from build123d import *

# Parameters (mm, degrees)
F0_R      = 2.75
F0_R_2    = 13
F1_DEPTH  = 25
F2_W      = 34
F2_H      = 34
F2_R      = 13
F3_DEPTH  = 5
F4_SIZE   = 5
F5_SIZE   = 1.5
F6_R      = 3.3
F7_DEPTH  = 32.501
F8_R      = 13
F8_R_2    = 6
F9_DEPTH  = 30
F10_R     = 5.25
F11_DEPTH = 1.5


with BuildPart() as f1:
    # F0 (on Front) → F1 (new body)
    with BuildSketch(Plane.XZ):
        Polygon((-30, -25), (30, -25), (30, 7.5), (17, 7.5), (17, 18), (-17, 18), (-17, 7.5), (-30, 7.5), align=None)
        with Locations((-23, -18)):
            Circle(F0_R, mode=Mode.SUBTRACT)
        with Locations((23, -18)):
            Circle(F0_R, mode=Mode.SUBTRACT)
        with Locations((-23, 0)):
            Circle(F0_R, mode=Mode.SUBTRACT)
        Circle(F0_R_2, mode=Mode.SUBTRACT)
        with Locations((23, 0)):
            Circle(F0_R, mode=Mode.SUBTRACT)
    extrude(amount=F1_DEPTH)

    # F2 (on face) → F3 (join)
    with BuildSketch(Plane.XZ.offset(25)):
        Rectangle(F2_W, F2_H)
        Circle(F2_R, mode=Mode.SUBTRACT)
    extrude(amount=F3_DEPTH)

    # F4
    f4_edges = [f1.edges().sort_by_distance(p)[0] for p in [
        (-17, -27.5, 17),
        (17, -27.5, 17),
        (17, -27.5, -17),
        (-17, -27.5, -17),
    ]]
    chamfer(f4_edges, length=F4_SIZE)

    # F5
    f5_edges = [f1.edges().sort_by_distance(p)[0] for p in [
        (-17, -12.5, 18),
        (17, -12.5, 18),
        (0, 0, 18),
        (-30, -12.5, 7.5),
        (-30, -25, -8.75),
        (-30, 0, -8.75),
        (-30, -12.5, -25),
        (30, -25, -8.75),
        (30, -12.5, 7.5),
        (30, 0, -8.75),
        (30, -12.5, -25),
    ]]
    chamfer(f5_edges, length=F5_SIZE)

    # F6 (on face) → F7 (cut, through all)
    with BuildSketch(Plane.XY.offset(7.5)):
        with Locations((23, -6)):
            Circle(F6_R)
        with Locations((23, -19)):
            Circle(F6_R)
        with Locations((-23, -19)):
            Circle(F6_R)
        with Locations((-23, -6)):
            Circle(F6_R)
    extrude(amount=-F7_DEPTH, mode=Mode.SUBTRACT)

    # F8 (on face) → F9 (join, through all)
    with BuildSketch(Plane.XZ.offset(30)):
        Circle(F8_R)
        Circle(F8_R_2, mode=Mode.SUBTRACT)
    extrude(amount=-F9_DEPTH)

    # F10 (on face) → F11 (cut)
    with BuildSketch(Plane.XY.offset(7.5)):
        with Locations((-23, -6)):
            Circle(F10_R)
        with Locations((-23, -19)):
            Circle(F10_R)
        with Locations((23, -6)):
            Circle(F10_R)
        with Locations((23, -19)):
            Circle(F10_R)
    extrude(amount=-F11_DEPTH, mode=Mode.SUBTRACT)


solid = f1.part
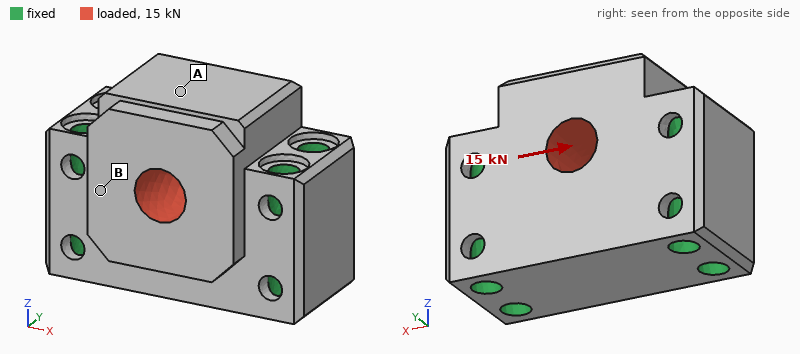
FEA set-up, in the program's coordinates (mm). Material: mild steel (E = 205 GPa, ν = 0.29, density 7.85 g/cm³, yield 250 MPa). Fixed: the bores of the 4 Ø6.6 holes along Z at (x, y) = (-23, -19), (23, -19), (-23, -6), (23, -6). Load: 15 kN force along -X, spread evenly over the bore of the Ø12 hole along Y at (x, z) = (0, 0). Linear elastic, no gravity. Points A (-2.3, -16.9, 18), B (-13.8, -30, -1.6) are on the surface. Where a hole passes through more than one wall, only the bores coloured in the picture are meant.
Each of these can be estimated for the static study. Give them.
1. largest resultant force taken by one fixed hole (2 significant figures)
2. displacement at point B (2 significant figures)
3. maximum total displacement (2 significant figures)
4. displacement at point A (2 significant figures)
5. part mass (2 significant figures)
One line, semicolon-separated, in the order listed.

4.2 kN; 1.1 µm; 1.8 µm; 0.99 µm; 420 g
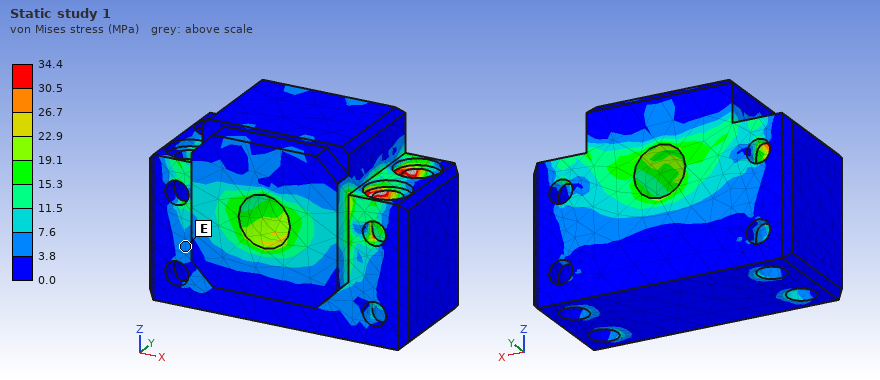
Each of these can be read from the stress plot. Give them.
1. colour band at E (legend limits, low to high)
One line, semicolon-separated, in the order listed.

3.8 to 7.6 MPa
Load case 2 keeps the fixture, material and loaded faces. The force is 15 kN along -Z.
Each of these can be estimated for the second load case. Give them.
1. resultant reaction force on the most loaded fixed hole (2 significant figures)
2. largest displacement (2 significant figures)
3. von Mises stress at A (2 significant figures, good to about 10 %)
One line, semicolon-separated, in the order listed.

4.5 kN; 3.2 µm; 15 MPa
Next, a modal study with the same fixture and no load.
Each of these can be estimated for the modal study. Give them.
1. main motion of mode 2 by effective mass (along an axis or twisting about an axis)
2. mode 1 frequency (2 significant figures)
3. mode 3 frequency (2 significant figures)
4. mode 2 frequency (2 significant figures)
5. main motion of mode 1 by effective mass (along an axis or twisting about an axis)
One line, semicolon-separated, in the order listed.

along Z; 20 kHz; 32 kHz; 30 kHz; along Y
